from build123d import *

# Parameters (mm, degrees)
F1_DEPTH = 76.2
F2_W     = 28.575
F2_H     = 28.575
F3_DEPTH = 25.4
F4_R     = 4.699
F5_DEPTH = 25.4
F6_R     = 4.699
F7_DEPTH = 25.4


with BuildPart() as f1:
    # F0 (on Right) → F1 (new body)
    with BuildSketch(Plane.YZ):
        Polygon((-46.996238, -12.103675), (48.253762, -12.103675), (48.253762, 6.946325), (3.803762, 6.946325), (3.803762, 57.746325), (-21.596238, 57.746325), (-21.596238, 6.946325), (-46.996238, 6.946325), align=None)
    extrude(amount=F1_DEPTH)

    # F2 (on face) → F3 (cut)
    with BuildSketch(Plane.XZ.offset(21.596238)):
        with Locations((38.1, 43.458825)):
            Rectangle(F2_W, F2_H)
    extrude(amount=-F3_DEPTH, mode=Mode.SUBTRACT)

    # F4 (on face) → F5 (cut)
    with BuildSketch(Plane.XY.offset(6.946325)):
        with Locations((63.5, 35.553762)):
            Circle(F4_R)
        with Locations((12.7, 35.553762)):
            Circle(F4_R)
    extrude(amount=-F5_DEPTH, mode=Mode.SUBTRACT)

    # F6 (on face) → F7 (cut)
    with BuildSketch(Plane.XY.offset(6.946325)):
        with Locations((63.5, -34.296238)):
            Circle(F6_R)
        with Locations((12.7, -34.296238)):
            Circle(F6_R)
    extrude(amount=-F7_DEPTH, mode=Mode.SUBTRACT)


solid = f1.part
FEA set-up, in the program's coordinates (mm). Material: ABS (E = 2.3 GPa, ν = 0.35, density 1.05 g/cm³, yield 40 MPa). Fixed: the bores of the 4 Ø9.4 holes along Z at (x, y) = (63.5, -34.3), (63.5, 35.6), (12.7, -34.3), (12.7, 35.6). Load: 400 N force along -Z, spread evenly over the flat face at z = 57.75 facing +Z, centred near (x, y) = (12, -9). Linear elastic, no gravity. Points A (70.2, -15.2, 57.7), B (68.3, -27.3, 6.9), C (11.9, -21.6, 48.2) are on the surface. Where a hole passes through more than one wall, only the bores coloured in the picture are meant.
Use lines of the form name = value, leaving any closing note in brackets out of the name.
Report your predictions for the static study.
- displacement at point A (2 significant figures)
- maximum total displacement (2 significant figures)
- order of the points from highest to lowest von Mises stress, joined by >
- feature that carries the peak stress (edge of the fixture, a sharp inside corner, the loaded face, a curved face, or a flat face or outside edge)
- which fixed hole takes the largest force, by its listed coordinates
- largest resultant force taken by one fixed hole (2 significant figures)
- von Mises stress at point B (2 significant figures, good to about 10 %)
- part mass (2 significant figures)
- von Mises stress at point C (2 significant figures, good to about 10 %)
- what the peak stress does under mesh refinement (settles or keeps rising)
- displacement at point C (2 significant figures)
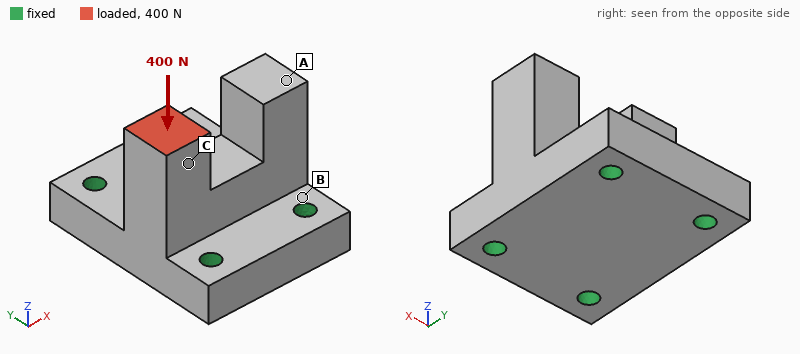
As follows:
displacement at point A = 16 µm
maximum total displacement = 49 µm
order of the points from highest to lowest von Mises stress, joined by > = C > B > A
feature that carries the peak stress = edge of the fixture
which fixed hole takes the largest force, by its listed coordinates = (12.7, -34.3)
largest resultant force taken by one fixed hole = 260 N
von Mises stress at point B = 0.33 MPa
part mass = 220 g
von Mises stress at point C = 0.66 MPa
what the peak stress does under mesh refinement = keeps rising
displacement at point C = 35 µm
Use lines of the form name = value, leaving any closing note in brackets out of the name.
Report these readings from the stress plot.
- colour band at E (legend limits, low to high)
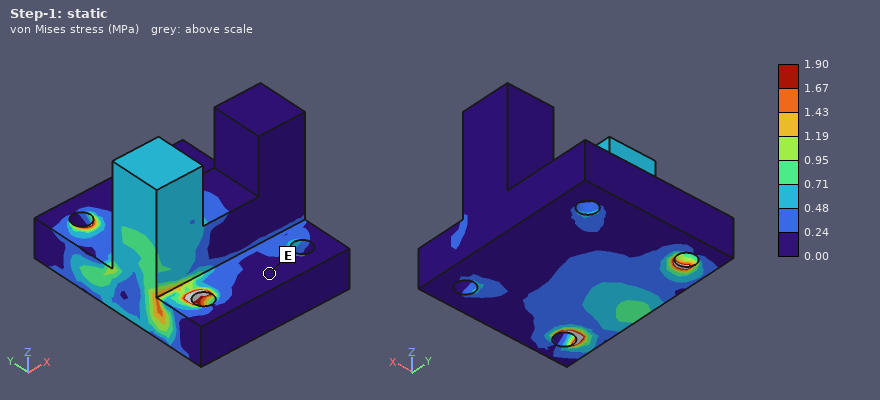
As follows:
colour band at E = 0.00 to 0.24 MPa
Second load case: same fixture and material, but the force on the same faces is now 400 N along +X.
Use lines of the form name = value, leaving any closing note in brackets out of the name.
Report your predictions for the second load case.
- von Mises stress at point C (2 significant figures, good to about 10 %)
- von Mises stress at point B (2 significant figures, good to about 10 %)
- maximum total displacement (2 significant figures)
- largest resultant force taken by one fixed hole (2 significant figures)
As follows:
von Mises stress at point C = 2.0 MPa
von Mises stress at point B = 1.7 MPa
maximum total displacement = 0.25 mm
largest resultant force taken by one fixed hole = 350 N
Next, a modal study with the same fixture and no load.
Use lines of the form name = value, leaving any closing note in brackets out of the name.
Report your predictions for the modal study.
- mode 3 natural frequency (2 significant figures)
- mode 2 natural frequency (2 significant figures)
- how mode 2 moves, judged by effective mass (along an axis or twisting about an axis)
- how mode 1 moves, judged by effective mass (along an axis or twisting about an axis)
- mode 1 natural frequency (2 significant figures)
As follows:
mode 3 natural frequency = 2000 Hz
mode 2 natural frequency = 1700 Hz
how mode 2 moves, judged by effective mass = along X
how mode 1 moves, judged by effective mass = along Y
mode 1 natural frequency = 1600 Hz
